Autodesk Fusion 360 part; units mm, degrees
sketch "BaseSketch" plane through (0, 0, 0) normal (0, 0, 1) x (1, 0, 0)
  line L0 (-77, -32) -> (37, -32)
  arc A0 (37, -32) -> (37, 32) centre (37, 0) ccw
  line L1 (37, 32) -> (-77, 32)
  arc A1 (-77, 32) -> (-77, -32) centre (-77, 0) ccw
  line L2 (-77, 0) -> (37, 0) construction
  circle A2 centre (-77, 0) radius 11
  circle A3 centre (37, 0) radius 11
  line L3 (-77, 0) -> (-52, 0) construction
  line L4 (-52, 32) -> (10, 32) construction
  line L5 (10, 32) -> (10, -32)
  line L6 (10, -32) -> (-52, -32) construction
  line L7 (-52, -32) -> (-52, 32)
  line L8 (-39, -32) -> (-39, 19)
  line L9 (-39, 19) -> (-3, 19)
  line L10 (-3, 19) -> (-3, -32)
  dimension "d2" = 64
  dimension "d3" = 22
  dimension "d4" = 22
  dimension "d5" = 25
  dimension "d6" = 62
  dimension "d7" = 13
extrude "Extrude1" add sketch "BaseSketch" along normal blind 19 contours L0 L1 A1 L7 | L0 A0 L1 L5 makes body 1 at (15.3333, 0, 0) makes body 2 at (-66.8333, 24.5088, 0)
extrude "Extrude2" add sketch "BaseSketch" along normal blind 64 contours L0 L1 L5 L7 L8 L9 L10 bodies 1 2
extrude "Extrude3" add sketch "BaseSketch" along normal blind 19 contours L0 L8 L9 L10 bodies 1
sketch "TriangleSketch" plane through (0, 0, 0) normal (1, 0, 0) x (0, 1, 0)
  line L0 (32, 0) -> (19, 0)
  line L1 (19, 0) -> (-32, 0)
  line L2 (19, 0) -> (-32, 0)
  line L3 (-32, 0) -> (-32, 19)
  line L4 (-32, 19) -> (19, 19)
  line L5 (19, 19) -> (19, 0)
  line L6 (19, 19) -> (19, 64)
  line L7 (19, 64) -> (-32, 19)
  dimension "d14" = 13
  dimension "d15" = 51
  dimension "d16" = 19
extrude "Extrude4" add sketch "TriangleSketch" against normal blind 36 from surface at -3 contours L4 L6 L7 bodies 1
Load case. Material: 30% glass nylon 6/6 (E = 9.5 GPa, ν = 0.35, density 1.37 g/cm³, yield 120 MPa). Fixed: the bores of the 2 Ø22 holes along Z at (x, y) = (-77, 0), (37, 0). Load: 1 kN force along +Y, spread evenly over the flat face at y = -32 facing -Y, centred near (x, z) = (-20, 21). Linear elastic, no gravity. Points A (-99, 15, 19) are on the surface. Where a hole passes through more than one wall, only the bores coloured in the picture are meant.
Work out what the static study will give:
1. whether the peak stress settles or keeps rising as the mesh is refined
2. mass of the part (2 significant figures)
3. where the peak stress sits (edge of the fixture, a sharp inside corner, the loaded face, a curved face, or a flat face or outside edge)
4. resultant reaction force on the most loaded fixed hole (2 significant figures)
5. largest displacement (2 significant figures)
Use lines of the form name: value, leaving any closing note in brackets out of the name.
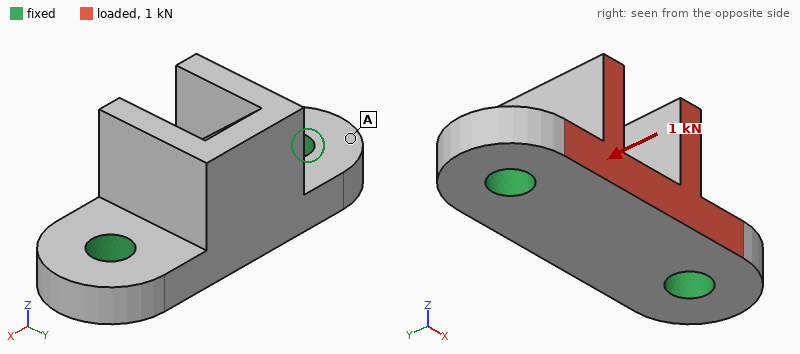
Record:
whether the peak stress settles or keeps rising as the mesh is refined: keeps rising
mass of the part: 440 g
where the peak stress sits: edge of the fixture
resultant reaction force on the most loaded fixed hole: 510 N
largest displacement: 22 µm
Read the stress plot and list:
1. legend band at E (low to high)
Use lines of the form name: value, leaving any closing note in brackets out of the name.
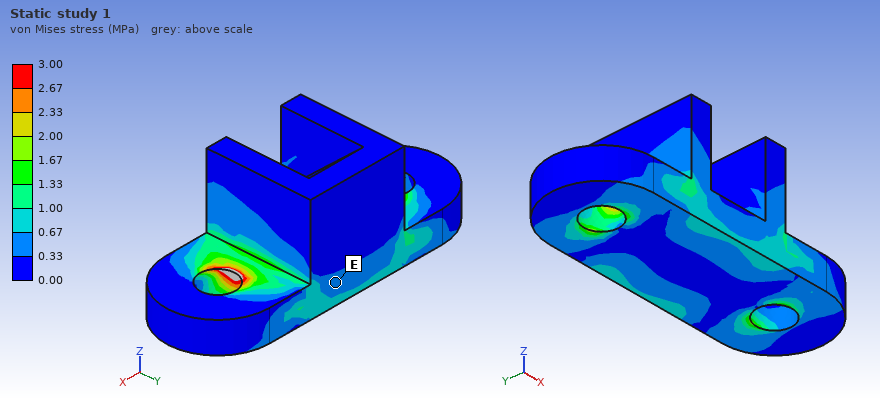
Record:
legend band at E: 0.33 to 0.67 MPa
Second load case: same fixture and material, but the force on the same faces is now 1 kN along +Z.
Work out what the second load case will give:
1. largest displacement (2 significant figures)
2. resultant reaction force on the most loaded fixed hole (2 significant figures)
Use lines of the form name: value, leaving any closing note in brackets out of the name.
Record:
largest displacement: 45 µm
resultant reaction force on the most loaded fixed hole: 520 N
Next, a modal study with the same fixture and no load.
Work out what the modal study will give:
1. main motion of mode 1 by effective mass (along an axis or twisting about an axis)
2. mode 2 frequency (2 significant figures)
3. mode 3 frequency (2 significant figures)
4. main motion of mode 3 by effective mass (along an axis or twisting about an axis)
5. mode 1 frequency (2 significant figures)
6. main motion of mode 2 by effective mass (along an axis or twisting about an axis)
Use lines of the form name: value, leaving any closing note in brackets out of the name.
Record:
main motion of mode 1 by effective mass: along Y
mode 2 frequency: 3200 Hz
mode 3 frequency: 3600 Hz
main motion of mode 3 by effective mass: along X
mode 1 frequency: 1800 Hz
main motion of mode 2 by effective mass: along Z
